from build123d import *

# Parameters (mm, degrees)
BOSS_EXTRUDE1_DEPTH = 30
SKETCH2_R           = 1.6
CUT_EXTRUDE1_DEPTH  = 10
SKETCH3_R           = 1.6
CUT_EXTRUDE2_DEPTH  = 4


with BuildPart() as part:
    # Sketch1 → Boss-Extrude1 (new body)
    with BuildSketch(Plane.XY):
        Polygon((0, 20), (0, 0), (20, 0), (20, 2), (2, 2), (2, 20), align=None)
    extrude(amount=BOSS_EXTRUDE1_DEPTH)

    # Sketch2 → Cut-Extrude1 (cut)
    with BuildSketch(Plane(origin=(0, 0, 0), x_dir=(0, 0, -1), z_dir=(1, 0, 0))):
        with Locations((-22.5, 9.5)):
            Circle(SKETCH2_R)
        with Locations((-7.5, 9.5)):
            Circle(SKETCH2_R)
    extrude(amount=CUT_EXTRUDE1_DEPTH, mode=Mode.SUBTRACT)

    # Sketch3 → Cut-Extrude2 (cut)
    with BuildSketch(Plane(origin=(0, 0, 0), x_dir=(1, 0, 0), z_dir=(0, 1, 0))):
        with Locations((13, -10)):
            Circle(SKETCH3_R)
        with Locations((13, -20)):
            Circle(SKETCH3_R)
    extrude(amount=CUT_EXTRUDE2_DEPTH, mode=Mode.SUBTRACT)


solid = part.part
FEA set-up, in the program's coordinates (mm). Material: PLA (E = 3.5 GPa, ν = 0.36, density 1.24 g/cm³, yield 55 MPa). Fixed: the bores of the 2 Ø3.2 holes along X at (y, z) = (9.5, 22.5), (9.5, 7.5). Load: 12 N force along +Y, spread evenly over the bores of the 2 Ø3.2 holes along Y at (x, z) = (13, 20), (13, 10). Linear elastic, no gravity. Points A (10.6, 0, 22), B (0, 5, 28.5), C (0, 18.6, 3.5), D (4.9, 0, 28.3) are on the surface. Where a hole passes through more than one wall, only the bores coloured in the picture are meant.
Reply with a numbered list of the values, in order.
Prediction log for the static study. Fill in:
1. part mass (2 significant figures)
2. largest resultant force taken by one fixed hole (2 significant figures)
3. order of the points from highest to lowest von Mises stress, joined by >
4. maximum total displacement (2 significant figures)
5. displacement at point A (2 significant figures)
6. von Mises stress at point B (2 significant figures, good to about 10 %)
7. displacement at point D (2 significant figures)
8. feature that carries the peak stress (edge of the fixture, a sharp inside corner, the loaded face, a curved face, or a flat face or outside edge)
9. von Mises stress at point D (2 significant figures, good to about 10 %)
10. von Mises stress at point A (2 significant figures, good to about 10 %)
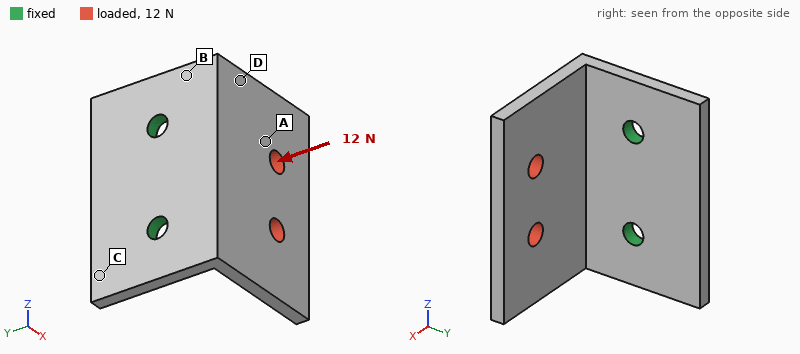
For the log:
1. 2.7 g
2. 6.2 N
3. B > D > A > C
4. 0.46 mm
5. 0.22 mm
6. 6.0 MPa
7. 0.10 mm
8. a flat face or outside edge
9. 4.5 MPa
10. 1.8 MPa
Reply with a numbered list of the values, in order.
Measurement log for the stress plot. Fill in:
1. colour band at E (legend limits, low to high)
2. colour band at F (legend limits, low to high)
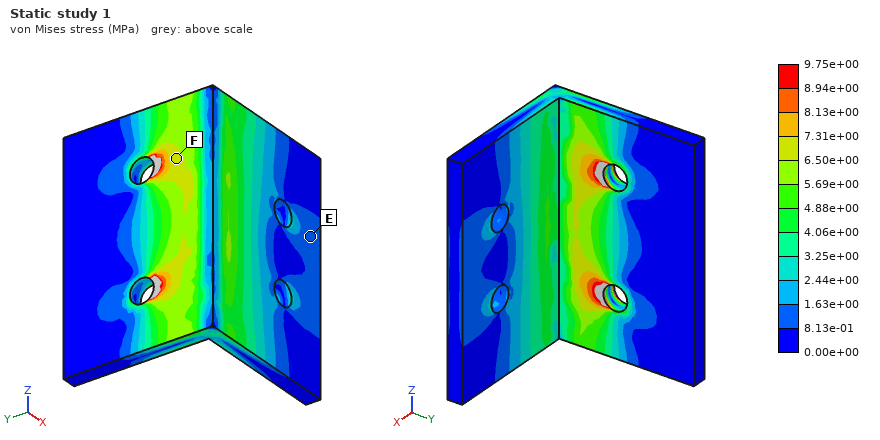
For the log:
1. 8.13e-01 to 1.63e+00 MPa
2. 6.50e+00 to 7.31e+00 MPa
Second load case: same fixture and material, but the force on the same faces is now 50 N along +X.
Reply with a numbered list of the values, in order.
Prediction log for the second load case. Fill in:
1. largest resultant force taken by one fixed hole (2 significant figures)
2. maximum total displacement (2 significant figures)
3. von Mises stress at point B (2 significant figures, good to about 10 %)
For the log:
1. 25 N
2. 0.45 mm
3. 7.9 MPa
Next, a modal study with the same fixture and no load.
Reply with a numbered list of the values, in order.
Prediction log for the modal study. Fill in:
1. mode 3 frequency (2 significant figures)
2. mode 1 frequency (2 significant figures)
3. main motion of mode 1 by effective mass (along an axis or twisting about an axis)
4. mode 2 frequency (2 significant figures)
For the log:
1. 2700 Hz
2. 950 Hz
3. along Y
4. 1800 Hz
